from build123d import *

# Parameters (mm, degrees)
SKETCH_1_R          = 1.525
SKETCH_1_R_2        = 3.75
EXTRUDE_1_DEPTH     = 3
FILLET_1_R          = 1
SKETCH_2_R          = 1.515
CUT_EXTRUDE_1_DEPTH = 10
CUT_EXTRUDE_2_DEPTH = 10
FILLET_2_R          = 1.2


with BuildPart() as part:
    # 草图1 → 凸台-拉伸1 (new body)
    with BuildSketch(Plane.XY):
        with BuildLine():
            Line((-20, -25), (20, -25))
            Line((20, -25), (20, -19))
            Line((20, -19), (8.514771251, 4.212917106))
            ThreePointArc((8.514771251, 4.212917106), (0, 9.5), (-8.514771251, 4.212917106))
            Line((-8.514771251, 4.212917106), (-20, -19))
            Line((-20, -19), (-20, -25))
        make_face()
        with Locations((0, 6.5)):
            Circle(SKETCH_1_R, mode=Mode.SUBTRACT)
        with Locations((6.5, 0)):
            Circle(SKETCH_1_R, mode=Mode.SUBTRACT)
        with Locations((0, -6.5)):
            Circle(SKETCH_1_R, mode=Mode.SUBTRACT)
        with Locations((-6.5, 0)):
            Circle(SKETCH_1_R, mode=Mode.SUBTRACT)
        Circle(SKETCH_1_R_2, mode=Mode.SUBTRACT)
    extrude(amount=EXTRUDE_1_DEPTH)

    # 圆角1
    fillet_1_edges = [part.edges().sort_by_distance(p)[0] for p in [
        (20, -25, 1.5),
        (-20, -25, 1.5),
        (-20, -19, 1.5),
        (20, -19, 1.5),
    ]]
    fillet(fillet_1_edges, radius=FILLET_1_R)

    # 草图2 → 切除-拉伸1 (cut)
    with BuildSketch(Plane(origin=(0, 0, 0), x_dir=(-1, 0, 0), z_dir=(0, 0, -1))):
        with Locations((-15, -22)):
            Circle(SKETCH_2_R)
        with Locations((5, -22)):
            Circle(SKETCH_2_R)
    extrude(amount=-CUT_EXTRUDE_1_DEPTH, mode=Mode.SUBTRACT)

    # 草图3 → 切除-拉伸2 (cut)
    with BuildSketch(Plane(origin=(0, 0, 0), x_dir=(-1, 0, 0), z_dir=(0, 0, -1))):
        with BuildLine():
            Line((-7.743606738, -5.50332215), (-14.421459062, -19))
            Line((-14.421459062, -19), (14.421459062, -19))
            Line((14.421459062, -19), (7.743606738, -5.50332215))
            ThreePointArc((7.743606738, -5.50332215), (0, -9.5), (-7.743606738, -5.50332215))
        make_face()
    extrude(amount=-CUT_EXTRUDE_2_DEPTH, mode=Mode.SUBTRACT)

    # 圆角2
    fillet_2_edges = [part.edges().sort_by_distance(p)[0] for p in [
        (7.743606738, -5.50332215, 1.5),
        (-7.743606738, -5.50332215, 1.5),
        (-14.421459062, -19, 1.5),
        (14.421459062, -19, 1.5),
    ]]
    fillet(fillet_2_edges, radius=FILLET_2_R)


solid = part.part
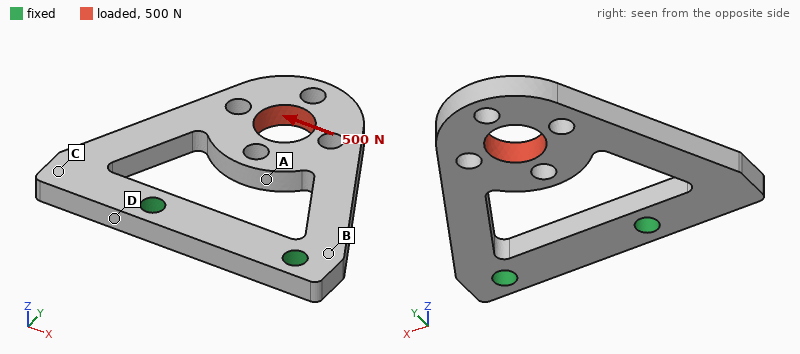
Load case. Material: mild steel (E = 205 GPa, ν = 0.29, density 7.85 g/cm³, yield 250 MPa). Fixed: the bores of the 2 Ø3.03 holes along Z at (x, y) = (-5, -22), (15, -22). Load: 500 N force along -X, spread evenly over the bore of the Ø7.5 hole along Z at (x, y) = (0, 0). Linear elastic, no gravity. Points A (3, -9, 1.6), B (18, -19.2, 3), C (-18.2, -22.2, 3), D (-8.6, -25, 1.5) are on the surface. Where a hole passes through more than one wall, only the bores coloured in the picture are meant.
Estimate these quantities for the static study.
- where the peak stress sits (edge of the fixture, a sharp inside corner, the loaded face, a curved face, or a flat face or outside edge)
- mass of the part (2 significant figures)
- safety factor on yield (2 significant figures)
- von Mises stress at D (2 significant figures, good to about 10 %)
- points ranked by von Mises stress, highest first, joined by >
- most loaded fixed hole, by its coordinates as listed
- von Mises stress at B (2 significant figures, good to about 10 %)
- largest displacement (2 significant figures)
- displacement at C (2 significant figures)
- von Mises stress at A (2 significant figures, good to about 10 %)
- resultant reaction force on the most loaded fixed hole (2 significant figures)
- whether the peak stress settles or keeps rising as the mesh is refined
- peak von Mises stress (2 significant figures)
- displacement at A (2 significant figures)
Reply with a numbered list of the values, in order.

1. a curved face
2. 15 g
3. 0.99
4. 110 MPa
5. D > B > A > C
6. (15, -22)
7. 68 MPa
8. 30 µm
9. 18 µm
10. 32 MPa
11. 430 N
12. settles
13. 250 MPa
14. 27 µm
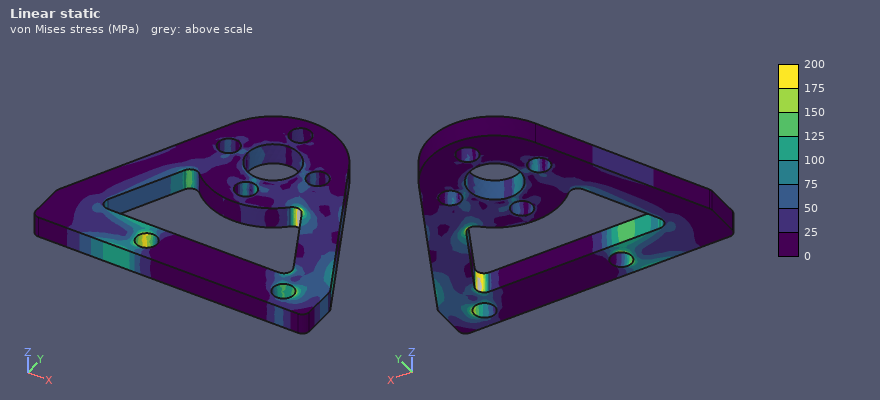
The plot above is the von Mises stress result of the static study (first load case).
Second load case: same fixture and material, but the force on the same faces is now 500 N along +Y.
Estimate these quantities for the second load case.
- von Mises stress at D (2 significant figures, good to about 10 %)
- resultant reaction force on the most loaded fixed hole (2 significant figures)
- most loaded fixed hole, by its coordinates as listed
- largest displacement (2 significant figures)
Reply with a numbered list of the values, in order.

1. 74 MPa
2. 280 N
3. (-5, -22)
4. 14 µm
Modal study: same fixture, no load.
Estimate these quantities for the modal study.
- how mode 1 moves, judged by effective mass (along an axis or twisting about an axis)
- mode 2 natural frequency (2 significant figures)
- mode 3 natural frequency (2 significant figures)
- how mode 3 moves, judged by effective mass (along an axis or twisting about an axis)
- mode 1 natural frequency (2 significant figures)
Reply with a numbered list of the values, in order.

1. along Z
2. 6500 Hz
3. 7300 Hz
4. along X
5. 2000 Hz
